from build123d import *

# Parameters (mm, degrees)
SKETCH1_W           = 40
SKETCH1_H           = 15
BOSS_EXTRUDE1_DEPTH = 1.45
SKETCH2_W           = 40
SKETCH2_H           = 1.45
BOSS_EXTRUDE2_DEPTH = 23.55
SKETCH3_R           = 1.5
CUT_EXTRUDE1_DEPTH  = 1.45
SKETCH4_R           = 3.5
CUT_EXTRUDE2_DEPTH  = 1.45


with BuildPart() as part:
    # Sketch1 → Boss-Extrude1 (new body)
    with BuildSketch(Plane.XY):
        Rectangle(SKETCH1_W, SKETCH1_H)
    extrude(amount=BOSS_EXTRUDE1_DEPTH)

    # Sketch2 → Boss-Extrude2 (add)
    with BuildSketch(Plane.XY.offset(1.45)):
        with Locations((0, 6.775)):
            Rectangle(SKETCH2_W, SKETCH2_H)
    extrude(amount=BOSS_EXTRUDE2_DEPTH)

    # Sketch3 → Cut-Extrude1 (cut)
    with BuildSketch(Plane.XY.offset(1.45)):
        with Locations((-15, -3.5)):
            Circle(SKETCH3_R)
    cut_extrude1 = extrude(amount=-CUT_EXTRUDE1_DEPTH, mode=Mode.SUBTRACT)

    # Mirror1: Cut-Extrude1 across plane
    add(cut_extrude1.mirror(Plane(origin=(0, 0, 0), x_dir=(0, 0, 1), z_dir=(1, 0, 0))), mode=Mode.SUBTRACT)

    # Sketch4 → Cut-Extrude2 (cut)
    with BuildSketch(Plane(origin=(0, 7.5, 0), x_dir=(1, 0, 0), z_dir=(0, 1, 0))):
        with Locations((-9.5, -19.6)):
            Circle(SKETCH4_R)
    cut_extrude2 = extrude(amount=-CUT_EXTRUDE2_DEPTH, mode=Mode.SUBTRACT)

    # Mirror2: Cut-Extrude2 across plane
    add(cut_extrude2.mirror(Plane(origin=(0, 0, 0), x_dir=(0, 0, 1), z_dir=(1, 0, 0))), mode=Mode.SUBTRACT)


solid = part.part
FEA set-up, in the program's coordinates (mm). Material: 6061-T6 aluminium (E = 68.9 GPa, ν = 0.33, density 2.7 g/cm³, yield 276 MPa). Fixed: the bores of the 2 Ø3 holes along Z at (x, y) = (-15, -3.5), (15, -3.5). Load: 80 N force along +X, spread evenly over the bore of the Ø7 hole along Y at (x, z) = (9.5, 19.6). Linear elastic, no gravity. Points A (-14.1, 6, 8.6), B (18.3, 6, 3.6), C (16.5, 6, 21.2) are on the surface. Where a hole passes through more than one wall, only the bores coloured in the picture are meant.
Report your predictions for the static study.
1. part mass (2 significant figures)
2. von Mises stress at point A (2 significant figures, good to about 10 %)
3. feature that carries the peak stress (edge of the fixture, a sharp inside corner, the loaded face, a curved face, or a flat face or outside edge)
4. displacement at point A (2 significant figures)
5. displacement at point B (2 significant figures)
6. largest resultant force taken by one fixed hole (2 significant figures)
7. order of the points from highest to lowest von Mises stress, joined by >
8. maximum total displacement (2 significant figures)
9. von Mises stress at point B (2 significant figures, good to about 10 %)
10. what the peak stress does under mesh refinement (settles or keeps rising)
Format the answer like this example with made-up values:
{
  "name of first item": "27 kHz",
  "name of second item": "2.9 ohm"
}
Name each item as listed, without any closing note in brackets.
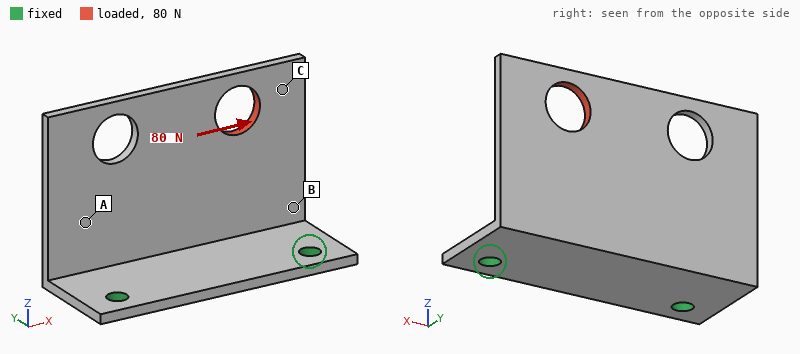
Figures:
{
  "part mass": "5.7 g",
  "von Mises stress at point A": "14 MPa",
  "feature that carries the peak stress": "edge of the fixture",
  "displacement at point A": "0.046 mm",
  "displacement at point B": "0.045 mm",
  "largest resultant force taken by one fixed hole": "68 N",
  "order of the points from highest to lowest von Mises stress, joined by >": "B > A > C",
  "maximum total displacement": "0.10 mm",
  "von Mises stress at point B": "28 MPa",
  "what the peak stress does under mesh refinement": "keeps rising"
}
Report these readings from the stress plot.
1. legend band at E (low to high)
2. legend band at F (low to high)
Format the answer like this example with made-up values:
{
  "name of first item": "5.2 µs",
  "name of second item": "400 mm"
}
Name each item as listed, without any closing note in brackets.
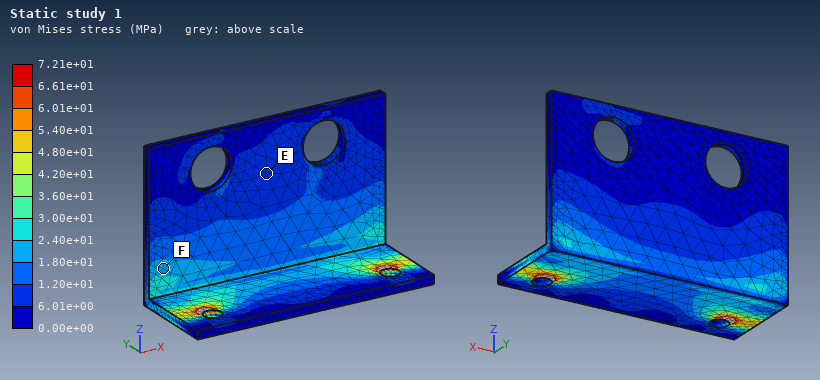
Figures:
{
  "legend band at E": "6.01e+00 to 1.20e+01 MPa",
  "legend band at F": "1.80e+01 to 2.40e+01 MPa"
}
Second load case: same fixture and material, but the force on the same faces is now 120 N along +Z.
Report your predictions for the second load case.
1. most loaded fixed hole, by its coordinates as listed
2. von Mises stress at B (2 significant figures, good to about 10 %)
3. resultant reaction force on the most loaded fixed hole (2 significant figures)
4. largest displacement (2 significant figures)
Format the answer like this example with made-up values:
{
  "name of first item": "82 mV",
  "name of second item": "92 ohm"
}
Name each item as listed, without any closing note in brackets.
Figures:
{
  "most loaded fixed hole, by its coordinates as listed": "(15, -3.5)",
  "von Mises stress at B": "33 MPa",
  "resultant reaction force on the most loaded fixed hole": "97 N",
  "largest displacement": "0.32 mm"
}
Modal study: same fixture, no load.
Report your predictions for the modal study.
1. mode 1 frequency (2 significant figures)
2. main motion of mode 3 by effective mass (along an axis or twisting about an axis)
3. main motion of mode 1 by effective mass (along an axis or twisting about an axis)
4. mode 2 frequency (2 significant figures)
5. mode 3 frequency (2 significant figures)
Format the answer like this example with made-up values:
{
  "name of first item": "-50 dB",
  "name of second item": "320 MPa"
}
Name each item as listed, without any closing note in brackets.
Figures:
{
  "mode 1 frequency": "1300 Hz",
  "main motion of mode 3 by effective mass": "along X",
  "main motion of mode 1 by effective mass": "along Y",
  "mode 2 frequency": "2700 Hz",
  "mode 3 frequency": "4400 Hz"
}
